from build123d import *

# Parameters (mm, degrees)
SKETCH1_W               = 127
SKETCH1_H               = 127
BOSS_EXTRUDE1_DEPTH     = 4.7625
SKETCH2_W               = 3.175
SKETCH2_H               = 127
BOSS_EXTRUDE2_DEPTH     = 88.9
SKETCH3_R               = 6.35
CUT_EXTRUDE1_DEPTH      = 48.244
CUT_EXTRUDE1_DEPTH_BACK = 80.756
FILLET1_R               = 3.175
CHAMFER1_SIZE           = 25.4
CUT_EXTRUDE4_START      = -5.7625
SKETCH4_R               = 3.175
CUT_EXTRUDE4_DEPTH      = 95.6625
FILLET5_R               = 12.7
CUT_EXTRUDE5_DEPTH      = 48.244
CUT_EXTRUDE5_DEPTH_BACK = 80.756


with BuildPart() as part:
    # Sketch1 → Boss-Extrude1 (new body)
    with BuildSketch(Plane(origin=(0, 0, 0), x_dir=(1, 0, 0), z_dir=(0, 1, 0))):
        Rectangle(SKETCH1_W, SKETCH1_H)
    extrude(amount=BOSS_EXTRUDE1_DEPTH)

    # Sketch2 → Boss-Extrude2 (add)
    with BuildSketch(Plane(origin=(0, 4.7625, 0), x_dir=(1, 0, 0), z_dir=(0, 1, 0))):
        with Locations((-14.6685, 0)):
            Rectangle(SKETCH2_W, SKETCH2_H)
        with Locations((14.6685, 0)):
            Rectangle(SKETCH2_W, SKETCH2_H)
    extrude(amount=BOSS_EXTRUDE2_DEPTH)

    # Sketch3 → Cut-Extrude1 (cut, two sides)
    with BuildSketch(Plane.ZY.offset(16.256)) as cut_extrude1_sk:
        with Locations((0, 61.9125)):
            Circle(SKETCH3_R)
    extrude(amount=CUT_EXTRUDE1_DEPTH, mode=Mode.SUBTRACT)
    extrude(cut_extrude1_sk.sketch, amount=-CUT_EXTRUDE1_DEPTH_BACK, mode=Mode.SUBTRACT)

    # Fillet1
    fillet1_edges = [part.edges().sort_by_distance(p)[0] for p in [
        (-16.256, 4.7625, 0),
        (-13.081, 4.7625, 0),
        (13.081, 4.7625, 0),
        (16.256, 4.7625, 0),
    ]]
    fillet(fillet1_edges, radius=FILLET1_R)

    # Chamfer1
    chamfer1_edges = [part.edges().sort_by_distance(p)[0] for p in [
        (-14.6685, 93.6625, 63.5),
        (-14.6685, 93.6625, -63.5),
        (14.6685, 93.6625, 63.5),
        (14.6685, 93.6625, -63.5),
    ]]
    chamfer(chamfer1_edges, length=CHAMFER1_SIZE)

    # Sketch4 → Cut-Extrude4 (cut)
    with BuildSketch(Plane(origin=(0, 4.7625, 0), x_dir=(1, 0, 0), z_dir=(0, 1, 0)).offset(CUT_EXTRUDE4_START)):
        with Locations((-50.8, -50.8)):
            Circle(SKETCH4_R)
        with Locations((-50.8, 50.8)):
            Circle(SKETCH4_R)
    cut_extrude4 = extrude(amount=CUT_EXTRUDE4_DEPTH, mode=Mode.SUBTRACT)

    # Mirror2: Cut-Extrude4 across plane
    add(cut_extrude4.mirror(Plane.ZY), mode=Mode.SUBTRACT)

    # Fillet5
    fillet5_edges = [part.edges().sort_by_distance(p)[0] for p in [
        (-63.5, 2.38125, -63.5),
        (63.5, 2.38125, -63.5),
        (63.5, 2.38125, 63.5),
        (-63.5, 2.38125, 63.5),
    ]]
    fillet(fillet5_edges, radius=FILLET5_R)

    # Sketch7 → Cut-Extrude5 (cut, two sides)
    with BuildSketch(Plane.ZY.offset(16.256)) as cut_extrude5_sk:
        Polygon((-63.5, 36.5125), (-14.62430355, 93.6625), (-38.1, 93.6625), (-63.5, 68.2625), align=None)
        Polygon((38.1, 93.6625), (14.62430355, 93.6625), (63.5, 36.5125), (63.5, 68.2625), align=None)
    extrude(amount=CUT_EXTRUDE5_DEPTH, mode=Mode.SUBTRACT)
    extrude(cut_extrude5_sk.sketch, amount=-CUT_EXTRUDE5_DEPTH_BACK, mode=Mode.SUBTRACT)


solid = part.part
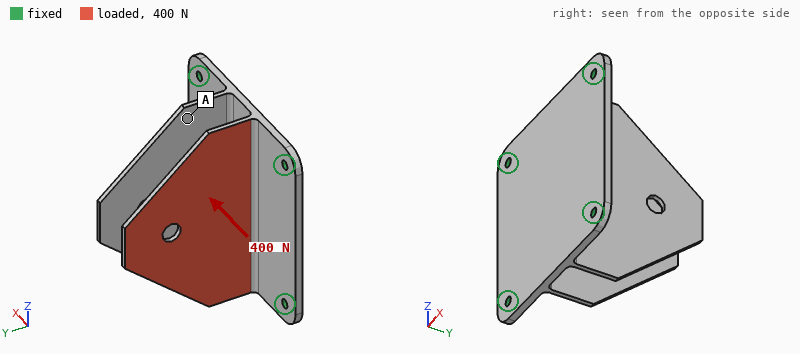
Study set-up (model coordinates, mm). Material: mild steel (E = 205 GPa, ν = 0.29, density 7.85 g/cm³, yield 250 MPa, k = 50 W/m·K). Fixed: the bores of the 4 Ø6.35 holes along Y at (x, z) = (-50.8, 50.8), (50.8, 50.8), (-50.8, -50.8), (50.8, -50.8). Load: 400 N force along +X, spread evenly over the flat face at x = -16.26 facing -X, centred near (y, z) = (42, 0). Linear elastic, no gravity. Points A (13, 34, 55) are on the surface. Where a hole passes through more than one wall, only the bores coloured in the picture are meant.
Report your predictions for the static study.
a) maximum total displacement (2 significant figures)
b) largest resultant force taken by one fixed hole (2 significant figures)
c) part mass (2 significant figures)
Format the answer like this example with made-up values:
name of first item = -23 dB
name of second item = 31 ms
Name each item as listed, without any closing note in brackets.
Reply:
maximum total displacement = 0.42 mm
largest resultant force taken by one fixed hole = 150 N
part mass = 1.0 kg
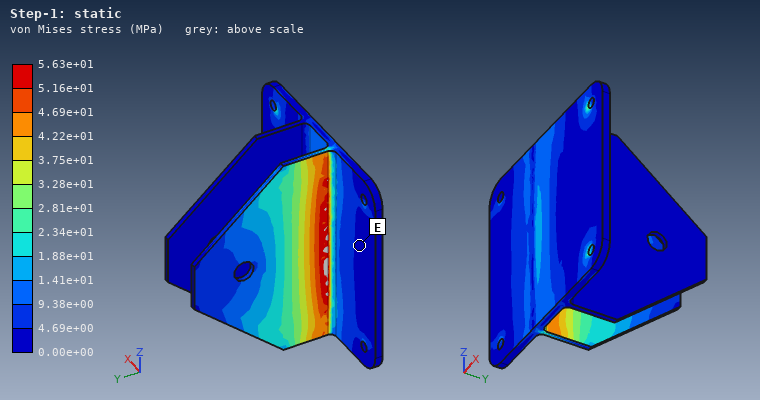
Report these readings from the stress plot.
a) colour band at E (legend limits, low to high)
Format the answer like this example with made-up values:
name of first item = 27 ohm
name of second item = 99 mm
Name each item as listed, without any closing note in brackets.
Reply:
colour band at E = 0.00e+00 to 4.69e+00 MPa
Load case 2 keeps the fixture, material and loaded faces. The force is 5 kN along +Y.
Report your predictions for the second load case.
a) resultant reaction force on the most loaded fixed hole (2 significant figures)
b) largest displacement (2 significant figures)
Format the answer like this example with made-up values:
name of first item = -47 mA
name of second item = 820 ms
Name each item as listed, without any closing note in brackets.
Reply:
resultant reaction force on the most loaded fixed hole = 1.8 kN
largest displacement = 0.25 mm
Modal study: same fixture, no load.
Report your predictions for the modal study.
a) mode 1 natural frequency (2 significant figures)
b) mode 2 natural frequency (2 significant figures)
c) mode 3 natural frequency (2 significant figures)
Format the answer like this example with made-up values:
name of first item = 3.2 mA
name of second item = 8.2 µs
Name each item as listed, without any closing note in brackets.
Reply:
mode 1 natural frequency = 460 Hz
mode 2 natural frequency = 480 Hz
mode 3 natural frequency = 1200 Hz
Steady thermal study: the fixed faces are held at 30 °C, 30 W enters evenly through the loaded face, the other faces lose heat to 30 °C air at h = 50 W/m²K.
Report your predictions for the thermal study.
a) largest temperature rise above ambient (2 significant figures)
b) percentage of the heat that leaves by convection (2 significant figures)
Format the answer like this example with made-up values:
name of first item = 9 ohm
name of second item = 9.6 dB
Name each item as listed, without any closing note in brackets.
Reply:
largest temperature rise above ambient = 41 K
percentage of the heat that leaves by convection = 78 %
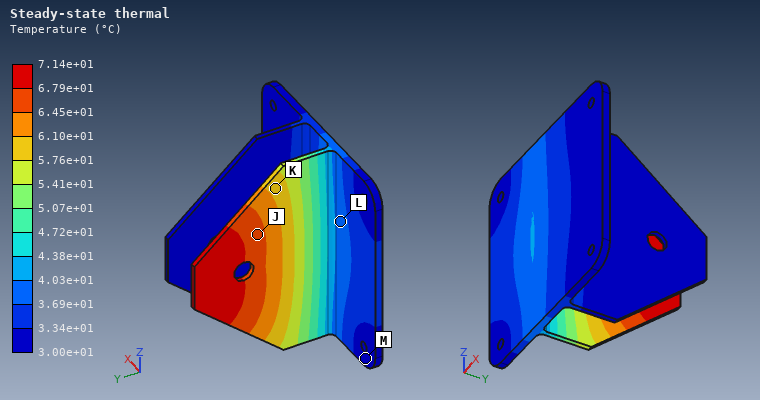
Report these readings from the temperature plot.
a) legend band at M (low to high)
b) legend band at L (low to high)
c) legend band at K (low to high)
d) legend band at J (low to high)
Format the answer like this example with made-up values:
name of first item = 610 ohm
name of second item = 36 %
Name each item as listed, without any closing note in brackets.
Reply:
legend band at M = 3.00e+01 to 3.34e+01 °C
legend band at L = 3.69e+01 to 4.03e+01 °C
legend band at K = 5.76e+01 to 6.10e+01 °C
legend band at J = 6.45e+01 to 6.79e+01 °C
